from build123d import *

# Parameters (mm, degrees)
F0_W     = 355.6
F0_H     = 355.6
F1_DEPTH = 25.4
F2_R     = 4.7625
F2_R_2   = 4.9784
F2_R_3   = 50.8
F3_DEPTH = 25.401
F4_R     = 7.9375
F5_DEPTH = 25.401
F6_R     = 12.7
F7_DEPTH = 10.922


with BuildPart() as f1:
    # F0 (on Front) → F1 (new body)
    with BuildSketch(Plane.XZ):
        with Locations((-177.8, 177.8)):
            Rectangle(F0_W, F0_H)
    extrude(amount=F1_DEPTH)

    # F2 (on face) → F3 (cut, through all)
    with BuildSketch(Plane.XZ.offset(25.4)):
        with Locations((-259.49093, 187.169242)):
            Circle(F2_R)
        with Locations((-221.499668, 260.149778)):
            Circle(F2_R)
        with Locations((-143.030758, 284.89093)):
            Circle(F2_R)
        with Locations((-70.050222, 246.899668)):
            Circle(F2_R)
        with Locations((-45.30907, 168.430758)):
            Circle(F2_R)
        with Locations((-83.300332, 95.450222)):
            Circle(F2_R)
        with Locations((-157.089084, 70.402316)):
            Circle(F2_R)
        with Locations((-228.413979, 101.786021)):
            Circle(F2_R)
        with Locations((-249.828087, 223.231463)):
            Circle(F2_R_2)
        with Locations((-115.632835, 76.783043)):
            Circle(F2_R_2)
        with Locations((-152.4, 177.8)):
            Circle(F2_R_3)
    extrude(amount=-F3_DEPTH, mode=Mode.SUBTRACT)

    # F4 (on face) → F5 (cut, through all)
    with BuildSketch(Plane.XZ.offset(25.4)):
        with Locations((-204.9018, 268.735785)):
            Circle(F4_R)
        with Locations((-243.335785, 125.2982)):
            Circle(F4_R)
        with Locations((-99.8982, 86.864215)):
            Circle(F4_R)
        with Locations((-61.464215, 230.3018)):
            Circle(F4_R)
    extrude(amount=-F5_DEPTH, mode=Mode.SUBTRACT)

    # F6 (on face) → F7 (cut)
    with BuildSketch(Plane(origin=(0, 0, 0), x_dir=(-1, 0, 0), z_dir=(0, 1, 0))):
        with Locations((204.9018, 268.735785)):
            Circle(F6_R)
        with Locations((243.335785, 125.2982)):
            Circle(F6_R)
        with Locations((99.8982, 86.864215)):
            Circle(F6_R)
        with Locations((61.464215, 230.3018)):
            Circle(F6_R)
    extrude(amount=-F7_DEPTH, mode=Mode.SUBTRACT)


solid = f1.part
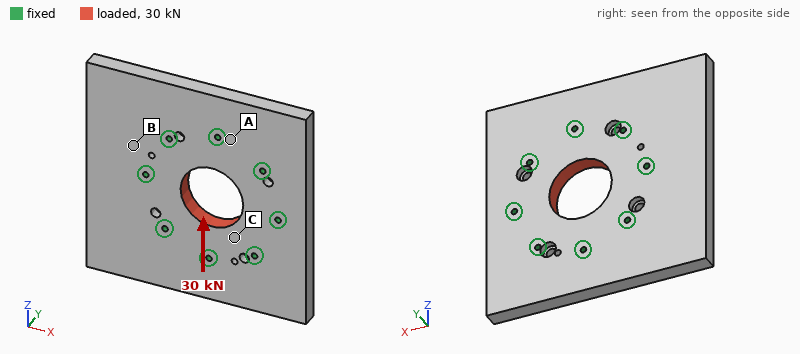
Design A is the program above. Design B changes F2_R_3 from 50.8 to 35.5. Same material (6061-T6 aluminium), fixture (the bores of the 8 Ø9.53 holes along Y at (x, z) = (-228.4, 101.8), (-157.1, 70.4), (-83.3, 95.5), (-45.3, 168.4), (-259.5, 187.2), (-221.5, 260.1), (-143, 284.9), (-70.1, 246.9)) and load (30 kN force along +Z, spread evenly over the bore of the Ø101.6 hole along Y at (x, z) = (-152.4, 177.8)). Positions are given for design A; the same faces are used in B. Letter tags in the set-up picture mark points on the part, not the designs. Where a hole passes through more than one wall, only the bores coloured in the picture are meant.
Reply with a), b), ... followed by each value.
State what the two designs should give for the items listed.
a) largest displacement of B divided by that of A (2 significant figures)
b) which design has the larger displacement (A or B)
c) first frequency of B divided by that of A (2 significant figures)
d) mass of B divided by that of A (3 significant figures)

a) 1.4
b) B
c) 1.0
d) 1.04
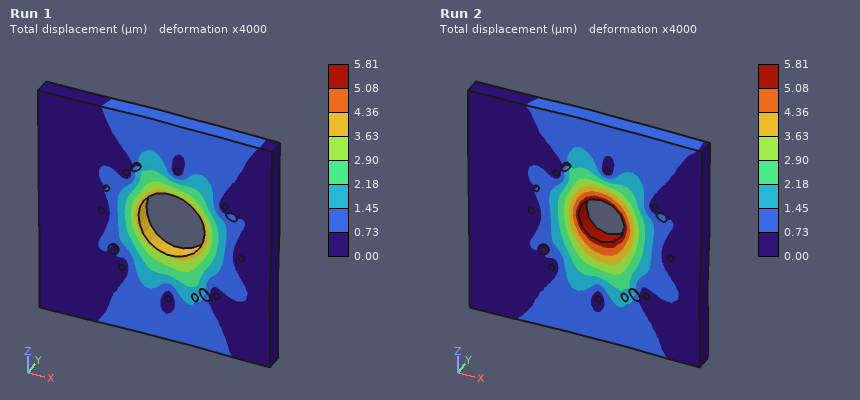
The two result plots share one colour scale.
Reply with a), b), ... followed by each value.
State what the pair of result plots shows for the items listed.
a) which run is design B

a) Run 2
